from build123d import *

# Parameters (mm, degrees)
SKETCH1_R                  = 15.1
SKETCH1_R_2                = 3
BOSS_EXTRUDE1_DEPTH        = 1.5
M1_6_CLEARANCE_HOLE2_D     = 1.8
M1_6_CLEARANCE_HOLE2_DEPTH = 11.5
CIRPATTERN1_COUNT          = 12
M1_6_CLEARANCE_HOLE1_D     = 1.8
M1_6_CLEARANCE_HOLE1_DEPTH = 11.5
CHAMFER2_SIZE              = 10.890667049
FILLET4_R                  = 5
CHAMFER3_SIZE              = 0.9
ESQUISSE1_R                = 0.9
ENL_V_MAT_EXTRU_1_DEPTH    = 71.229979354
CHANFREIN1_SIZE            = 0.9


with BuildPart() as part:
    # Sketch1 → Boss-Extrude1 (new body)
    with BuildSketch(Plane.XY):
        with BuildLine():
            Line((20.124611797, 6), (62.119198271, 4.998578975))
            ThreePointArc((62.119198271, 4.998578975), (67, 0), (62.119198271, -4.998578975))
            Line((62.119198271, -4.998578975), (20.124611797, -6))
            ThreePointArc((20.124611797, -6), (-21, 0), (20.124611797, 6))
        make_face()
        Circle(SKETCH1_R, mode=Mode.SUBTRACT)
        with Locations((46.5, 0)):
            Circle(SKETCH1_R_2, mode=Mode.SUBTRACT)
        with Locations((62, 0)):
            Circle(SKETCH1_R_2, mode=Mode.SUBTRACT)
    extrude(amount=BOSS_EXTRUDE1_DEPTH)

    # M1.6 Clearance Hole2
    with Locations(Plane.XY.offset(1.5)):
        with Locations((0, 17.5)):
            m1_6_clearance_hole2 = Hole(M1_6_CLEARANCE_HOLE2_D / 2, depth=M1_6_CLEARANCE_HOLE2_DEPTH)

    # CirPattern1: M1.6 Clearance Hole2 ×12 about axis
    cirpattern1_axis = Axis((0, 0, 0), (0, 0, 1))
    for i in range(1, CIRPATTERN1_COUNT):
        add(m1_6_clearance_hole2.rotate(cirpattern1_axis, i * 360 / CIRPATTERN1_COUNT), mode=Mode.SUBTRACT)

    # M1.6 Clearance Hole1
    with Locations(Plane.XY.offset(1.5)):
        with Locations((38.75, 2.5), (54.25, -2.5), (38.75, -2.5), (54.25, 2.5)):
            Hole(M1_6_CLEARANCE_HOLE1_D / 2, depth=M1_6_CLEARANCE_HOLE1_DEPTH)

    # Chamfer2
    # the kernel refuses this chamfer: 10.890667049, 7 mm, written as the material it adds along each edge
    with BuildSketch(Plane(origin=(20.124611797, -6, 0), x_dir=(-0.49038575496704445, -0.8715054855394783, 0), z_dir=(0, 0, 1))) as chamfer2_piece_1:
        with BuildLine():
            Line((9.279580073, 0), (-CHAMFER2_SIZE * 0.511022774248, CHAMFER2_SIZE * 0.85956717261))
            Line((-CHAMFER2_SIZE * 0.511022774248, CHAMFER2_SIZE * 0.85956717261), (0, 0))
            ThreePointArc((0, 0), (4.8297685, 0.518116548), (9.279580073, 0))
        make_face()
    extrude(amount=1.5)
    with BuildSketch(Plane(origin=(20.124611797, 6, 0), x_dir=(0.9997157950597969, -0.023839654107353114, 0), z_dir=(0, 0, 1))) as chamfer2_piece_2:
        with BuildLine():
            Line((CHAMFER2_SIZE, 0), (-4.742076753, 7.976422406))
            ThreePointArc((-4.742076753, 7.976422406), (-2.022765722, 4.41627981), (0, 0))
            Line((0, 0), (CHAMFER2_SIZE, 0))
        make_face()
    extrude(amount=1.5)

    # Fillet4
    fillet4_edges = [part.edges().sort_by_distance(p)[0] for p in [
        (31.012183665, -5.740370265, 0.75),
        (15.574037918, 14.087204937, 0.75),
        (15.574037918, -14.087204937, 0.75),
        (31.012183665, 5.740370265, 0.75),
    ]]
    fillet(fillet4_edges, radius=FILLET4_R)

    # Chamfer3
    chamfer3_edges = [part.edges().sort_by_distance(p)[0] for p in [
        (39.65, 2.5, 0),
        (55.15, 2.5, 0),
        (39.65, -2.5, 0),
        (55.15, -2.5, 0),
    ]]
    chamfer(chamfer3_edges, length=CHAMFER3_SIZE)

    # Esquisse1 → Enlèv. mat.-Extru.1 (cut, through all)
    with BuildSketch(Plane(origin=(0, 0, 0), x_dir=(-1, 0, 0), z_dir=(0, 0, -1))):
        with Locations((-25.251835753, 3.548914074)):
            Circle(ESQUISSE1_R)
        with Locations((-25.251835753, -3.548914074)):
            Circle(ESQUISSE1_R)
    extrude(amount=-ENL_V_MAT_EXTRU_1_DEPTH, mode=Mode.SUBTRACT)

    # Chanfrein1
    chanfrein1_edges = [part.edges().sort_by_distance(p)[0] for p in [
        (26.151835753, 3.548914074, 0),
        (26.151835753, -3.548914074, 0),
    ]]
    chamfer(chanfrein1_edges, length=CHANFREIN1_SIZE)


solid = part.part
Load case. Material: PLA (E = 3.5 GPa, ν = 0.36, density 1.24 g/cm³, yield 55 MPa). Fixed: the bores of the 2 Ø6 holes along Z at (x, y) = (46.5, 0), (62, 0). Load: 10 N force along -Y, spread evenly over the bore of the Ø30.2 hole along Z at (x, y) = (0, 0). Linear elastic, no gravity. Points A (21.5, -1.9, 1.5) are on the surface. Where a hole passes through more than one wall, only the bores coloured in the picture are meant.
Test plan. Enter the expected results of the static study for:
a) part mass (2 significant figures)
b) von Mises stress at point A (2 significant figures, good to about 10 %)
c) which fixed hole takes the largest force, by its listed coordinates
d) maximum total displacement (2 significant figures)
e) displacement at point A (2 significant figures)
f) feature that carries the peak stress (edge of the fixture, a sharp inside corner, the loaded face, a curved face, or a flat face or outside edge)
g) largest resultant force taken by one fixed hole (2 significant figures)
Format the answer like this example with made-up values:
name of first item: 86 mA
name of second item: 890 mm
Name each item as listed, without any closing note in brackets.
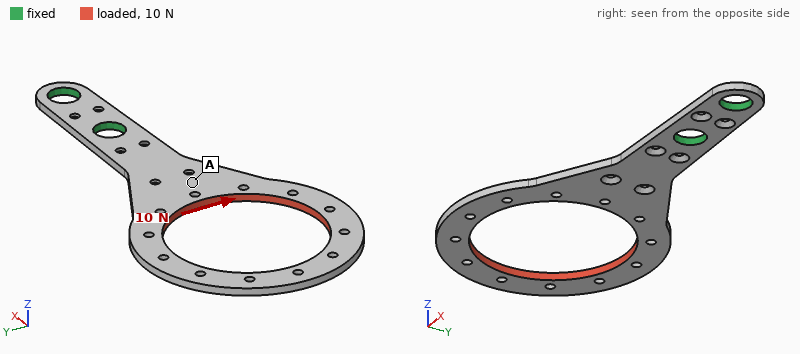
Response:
part mass: 2.1 g
von Mises stress at point A: 2.3 MPa
which fixed hole takes the largest force, by its listed coordinates: (46.5, 0)
maximum total displacement: 0.99 mm
displacement at point A: 0.24 mm
feature that carries the peak stress: a curved face
largest resultant force taken by one fixed hole: 13 N
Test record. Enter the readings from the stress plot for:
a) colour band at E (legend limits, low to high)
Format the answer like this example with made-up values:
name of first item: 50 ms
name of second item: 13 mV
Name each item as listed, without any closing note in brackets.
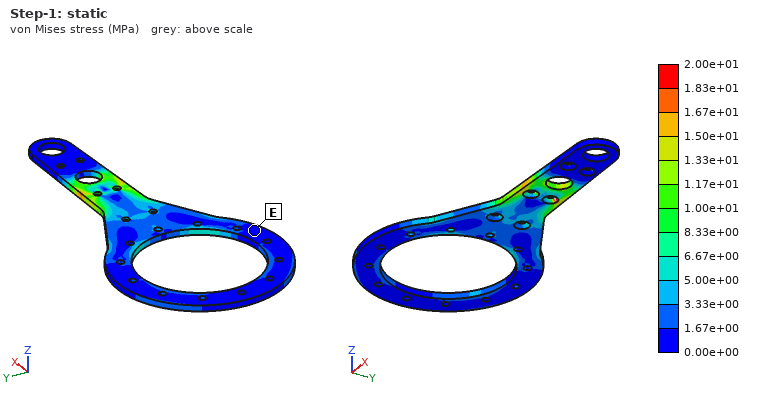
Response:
colour band at E: 0.00e+00 to 1.67e+00 MPa
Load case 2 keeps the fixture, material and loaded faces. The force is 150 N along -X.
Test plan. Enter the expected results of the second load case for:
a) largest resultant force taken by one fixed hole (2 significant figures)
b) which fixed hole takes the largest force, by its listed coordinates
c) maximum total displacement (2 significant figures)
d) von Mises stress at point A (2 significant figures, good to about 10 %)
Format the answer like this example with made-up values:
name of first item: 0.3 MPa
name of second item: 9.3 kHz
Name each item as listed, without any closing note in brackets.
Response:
largest resultant force taken by one fixed hole: 150 N
which fixed hole takes the largest force, by its listed coordinates: (46.5, 0)
maximum total displacement: 0.69 mm
von Mises stress at point A: 2.7 MPa
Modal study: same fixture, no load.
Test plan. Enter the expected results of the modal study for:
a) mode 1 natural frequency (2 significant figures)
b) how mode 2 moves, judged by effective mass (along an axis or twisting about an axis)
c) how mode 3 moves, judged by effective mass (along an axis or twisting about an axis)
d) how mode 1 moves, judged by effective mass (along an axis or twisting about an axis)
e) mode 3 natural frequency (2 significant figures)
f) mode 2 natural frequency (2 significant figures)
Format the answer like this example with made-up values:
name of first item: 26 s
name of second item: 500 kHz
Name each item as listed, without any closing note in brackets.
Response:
mode 1 natural frequency: 79 Hz
how mode 2 moves, judged by effective mass: twisting about X
how mode 3 moves, judged by effective mass: along Z
how mode 1 moves, judged by effective mass: along Z
mode 3 natural frequency: 460 Hz
mode 2 natural frequency: 230 Hz
